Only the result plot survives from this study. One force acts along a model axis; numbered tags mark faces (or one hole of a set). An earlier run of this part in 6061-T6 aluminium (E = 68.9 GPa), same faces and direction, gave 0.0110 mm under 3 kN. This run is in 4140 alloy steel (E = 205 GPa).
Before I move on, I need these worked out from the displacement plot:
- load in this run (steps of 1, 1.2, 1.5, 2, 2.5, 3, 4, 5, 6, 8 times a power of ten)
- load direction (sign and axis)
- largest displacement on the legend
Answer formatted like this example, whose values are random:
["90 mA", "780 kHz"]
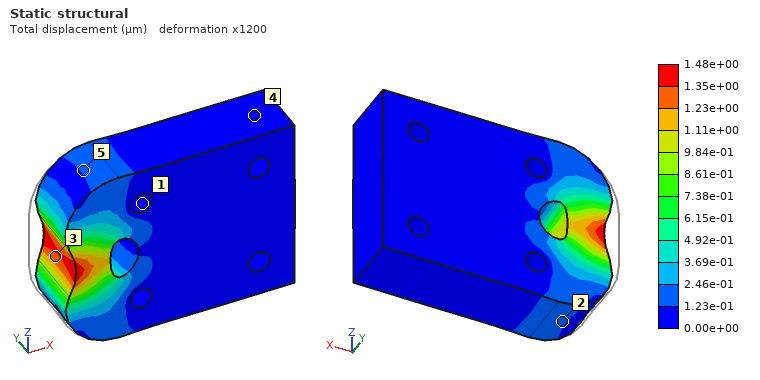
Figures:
["1.2 kN", "+X", "1.48e+00 µm"]
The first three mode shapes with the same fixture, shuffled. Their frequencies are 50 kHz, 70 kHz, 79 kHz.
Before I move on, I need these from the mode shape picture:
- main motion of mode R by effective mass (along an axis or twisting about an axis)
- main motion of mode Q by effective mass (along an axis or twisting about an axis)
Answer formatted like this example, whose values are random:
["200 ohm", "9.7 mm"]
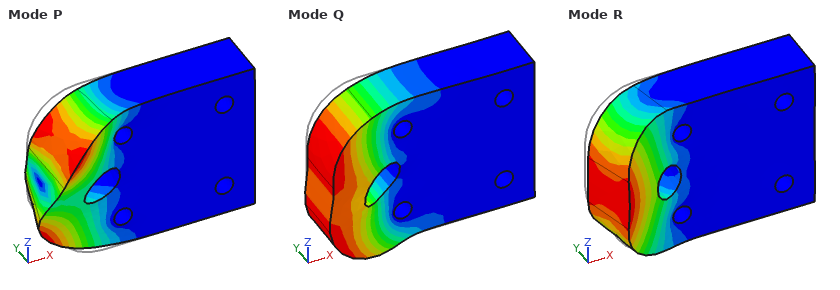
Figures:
["along Y", "along Z"]
